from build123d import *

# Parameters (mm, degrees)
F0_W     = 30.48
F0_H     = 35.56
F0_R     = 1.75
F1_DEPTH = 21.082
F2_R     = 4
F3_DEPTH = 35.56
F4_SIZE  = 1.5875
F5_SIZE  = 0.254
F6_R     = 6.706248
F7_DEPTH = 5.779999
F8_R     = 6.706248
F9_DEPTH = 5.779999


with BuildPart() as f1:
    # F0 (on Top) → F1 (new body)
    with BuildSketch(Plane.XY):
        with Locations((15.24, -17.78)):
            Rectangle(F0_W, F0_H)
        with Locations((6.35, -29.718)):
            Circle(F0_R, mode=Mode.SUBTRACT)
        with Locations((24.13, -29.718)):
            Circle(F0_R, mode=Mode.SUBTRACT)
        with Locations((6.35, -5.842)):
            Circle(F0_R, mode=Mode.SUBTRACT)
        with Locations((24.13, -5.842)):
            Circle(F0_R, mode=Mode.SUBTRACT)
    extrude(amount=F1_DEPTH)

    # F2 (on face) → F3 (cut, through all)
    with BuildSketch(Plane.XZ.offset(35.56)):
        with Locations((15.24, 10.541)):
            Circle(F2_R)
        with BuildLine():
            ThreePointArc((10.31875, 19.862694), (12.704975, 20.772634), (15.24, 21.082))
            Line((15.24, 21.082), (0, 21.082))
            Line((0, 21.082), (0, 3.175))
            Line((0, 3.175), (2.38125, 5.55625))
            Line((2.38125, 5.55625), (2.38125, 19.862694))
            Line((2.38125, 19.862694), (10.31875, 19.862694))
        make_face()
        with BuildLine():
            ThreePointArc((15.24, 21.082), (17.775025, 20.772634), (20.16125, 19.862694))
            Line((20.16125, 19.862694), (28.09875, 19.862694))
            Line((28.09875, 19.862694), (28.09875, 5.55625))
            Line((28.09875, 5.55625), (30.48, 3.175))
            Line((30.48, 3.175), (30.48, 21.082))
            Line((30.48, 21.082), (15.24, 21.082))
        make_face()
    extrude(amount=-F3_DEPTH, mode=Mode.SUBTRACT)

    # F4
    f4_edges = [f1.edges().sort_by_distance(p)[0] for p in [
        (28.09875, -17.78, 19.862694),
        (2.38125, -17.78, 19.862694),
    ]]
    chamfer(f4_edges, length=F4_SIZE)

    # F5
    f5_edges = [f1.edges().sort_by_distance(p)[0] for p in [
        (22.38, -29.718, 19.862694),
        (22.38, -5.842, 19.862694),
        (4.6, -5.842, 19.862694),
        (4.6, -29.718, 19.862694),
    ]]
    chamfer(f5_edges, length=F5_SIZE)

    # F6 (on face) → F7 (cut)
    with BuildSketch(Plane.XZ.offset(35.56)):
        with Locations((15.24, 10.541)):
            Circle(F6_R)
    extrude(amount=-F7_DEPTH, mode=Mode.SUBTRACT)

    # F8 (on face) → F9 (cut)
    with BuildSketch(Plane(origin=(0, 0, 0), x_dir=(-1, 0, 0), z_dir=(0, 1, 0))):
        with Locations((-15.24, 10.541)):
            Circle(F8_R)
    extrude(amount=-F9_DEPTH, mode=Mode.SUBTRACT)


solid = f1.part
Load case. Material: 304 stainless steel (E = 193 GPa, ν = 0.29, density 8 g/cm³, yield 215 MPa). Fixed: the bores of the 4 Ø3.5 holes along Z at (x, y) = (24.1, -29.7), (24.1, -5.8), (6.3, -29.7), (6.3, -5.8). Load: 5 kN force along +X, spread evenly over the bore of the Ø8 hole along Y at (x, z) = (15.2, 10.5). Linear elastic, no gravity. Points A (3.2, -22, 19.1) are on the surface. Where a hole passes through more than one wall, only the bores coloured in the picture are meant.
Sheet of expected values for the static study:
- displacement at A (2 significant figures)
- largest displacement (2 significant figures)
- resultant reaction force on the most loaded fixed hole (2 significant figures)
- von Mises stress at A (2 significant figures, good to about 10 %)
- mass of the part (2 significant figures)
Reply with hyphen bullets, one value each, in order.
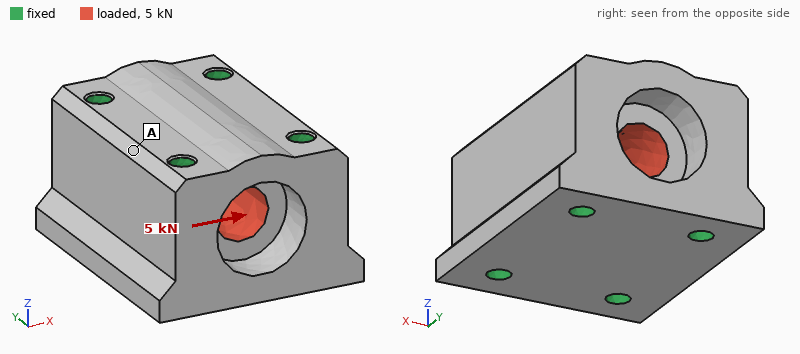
- 0.46 µm
- 0.75 µm
- 1.3 kN
- 4.0 MPa
- 120 g
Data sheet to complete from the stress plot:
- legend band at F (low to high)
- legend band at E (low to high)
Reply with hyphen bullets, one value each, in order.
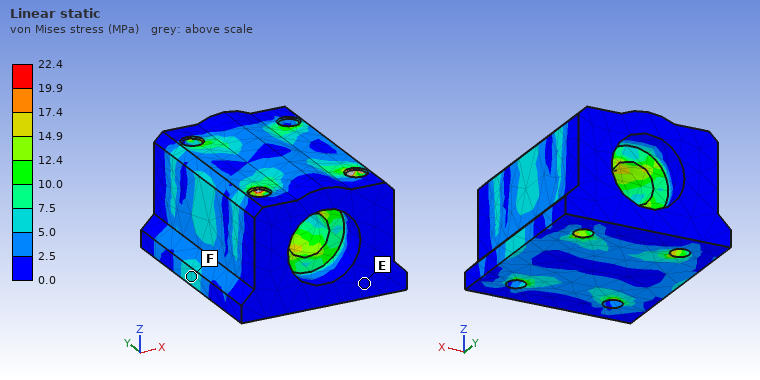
- 5.0 to 7.5 MPa
- 0.0 to 2.5 MPa
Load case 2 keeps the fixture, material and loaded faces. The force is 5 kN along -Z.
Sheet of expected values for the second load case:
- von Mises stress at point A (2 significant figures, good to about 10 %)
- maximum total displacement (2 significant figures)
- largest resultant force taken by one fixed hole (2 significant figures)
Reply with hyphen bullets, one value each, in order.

- 3.8 MPa
- 1.1 µm
- 1.3 kN
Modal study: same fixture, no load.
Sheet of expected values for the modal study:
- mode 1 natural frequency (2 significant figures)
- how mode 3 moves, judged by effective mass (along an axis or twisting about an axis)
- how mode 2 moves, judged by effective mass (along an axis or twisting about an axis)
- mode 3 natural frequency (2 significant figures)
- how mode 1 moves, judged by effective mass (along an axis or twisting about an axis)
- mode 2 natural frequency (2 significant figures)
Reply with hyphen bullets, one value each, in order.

- 53 kHz
- twisting about Y
- along X
- 60 kHz
- along Z
- 56 kHz
